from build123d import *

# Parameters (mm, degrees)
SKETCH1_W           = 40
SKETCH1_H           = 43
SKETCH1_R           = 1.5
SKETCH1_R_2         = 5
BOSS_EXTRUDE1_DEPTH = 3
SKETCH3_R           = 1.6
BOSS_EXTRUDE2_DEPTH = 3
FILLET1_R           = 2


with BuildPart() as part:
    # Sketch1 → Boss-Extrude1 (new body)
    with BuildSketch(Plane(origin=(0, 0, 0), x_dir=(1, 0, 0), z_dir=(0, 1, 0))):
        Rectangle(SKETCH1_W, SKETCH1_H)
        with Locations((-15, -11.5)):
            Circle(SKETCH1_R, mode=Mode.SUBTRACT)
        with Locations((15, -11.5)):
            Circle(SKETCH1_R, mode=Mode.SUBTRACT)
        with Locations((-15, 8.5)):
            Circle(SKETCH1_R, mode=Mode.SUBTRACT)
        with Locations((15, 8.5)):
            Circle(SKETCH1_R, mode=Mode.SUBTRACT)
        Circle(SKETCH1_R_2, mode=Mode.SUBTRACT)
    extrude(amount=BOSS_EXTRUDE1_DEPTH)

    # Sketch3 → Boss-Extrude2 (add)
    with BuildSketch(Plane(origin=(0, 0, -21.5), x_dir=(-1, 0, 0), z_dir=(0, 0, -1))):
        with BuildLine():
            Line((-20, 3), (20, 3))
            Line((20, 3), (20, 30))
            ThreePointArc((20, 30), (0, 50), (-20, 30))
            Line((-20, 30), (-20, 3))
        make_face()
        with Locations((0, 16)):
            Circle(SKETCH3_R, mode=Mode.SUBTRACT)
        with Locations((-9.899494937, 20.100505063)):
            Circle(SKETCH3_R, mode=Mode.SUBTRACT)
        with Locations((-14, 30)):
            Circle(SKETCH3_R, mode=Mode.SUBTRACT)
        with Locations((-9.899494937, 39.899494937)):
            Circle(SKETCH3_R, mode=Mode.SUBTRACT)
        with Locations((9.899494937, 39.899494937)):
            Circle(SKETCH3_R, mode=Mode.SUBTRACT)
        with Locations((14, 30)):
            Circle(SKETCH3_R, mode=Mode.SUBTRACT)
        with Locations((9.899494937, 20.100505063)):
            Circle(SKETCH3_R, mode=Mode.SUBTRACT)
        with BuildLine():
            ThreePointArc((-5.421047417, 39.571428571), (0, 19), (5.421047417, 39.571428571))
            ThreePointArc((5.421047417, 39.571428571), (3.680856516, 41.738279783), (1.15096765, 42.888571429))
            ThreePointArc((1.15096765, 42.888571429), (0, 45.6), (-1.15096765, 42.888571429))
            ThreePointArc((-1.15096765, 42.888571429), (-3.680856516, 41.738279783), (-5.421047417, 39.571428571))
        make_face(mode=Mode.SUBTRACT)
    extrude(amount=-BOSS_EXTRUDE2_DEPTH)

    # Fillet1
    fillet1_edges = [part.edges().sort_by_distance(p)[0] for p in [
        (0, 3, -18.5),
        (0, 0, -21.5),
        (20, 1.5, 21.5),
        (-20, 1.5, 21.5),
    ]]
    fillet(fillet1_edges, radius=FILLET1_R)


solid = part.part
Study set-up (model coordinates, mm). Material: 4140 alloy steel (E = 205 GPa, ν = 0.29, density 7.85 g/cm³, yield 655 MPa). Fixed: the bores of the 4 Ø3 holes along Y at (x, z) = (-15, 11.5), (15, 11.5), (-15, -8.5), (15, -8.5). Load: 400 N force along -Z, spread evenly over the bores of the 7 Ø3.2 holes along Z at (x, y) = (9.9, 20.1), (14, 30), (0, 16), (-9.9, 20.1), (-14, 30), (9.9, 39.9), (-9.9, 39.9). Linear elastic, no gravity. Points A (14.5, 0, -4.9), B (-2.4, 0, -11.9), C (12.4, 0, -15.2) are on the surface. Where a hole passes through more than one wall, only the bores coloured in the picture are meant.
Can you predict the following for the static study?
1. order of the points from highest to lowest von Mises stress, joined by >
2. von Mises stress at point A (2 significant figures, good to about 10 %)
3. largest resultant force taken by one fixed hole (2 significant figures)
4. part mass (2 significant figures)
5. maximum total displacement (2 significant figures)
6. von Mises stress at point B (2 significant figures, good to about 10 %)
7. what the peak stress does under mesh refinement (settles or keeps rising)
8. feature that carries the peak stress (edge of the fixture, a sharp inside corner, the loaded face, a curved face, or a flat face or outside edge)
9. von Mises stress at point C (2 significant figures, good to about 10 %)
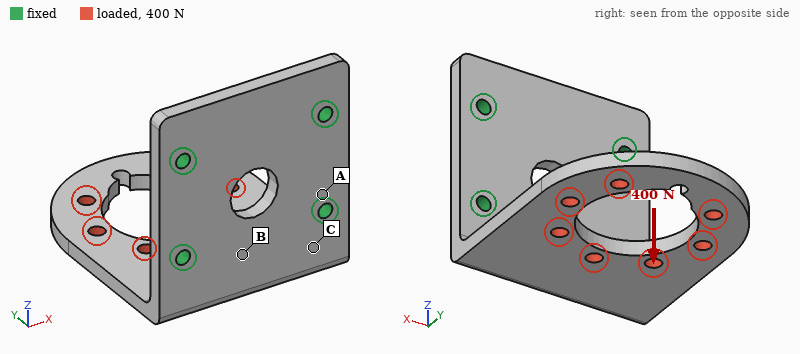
C > B > A
35 MPa
170 N
67 g
0.65 mm
110 MPa
keeps rising
edge of the fixture
160 MPa
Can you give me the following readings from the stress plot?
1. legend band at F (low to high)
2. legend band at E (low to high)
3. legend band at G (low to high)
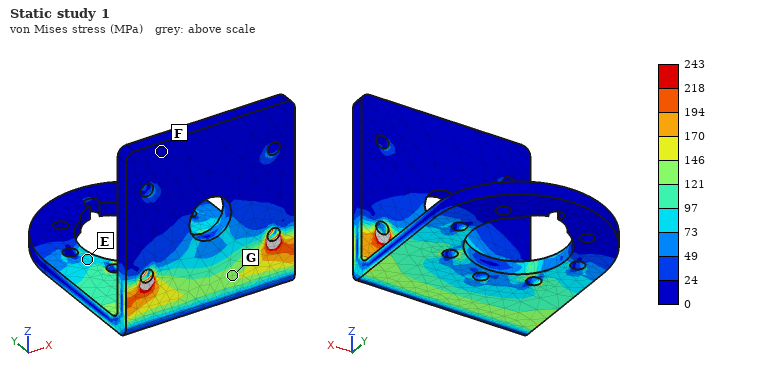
0 to 24 MPa
73 to 97 MPa
121 to 146 MPa
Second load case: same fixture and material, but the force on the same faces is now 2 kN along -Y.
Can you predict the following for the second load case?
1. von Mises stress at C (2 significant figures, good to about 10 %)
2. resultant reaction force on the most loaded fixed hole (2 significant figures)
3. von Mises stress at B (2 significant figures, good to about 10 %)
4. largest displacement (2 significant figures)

160 MPa
1.1 kN
130 MPa
0.39 mm
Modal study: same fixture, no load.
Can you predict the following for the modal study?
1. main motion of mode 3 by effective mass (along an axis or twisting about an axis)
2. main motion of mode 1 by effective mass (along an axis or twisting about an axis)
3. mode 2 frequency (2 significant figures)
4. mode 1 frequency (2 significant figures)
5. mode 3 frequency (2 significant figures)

along X
along Z
2800 Hz
1000 Hz
3900 Hz
